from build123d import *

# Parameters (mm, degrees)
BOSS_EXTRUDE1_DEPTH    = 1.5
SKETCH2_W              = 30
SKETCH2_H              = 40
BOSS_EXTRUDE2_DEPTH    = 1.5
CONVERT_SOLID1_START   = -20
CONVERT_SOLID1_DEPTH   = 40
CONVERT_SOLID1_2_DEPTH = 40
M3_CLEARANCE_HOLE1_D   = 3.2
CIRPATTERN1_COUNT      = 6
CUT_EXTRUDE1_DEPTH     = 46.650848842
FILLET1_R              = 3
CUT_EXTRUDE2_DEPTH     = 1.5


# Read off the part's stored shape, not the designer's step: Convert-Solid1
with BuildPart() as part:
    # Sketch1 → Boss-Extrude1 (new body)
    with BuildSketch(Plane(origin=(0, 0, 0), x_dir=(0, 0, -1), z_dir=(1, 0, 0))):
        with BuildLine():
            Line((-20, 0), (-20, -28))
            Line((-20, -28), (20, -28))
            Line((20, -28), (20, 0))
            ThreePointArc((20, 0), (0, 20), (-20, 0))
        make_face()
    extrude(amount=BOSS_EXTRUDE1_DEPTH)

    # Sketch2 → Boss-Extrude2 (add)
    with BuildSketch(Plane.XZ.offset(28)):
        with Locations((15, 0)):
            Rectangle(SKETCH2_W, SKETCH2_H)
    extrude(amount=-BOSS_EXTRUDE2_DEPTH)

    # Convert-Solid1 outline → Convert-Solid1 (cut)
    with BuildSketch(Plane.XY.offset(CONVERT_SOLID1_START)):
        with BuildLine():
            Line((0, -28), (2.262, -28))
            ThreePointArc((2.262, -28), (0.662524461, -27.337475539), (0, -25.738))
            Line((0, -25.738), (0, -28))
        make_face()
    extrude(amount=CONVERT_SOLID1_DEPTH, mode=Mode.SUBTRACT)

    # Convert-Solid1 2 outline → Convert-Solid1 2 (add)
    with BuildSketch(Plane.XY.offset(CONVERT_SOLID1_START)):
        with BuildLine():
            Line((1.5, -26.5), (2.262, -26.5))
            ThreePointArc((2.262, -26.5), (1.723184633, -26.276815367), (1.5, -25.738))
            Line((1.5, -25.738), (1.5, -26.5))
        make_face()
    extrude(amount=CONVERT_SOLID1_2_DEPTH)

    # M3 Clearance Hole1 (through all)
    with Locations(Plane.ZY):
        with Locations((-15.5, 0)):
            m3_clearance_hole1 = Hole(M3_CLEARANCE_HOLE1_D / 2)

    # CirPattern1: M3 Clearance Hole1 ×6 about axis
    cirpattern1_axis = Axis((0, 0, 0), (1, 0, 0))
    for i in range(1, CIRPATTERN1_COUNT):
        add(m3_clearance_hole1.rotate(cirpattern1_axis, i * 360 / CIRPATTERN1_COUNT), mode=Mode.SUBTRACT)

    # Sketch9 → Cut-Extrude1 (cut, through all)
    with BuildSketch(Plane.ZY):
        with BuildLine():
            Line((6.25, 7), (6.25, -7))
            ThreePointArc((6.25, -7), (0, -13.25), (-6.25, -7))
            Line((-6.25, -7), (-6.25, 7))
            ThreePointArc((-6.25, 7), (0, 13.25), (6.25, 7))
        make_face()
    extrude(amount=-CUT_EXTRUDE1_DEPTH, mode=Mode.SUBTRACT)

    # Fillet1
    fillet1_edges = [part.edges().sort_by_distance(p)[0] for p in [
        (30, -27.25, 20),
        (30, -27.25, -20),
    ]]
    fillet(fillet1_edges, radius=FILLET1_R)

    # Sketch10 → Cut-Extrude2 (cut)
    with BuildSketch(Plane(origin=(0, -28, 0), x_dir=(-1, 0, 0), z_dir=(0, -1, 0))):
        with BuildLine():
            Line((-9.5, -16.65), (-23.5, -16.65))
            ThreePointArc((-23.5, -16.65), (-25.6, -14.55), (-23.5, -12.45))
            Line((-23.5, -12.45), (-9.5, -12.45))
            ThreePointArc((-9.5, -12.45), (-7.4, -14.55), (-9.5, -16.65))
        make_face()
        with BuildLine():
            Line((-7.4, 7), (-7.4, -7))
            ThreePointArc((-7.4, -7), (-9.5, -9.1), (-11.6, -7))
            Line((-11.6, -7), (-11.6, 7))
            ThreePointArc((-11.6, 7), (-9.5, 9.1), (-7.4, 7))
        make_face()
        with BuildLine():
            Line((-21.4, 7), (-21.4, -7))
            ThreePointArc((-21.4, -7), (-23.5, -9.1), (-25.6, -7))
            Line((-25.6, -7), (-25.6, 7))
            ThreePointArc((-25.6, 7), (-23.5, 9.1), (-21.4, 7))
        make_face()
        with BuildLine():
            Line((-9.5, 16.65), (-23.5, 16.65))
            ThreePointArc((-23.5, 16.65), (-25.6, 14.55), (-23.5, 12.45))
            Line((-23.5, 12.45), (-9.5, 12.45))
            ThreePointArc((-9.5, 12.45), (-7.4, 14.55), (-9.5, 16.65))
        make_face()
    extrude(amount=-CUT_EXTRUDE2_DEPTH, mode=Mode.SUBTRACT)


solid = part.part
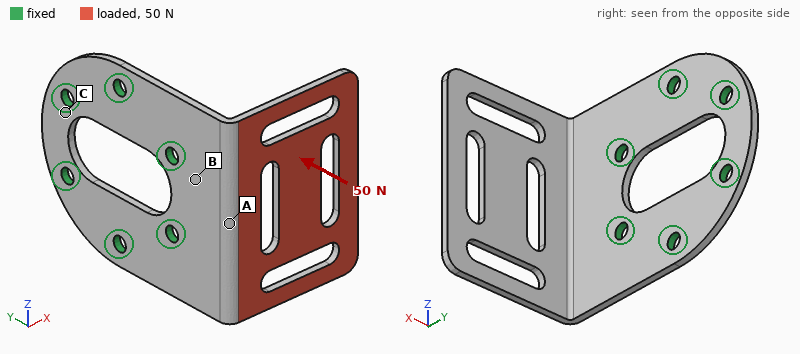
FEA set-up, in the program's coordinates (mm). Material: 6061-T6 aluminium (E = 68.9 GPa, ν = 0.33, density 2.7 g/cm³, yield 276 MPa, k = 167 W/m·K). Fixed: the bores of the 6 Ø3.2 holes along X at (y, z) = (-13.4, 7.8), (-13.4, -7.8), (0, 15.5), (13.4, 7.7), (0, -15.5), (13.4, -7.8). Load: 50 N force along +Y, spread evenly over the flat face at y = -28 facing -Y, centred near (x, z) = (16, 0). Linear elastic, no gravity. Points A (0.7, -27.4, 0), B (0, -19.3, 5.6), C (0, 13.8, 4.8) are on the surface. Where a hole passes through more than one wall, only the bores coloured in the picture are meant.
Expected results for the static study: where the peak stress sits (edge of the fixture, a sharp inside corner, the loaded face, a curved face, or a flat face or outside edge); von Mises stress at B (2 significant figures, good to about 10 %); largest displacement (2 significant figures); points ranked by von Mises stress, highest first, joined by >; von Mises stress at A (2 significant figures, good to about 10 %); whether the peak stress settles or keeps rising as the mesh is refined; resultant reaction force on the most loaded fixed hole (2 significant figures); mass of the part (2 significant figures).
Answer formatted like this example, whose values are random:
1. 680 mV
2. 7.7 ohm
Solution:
1. a sharp inside corner
2. 46 MPa
3. 0.75 mm
4. B > A > C
5. 21 MPa
6. keeps rising
7. 22 N
8. 9.0 g
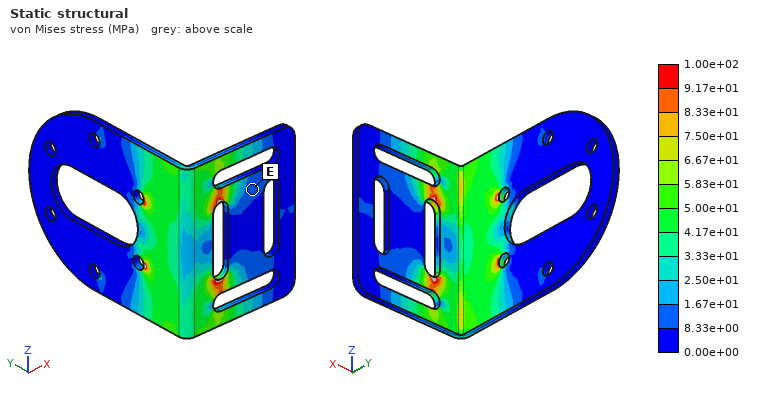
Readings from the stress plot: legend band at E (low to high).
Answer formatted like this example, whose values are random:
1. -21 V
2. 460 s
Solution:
1. 8.33e+00 to 1.67e+01 MPa
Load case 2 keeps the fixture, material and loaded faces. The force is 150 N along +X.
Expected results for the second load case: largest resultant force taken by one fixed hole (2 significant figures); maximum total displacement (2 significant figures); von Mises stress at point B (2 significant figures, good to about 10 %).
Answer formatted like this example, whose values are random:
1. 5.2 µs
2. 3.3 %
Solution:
1. 93 N
2. 0.67 mm
3. 88 MPa
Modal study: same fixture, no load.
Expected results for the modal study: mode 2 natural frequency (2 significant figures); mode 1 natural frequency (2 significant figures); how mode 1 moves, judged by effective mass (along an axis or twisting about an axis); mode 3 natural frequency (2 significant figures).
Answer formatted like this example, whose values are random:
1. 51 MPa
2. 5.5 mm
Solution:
1. 1700 Hz
2. 860 Hz
3. along Y
4. 2600 Hz
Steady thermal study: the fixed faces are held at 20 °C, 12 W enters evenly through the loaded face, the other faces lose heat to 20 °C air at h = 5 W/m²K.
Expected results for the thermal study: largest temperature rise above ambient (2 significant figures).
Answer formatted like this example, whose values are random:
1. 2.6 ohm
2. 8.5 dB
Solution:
1. 57 K
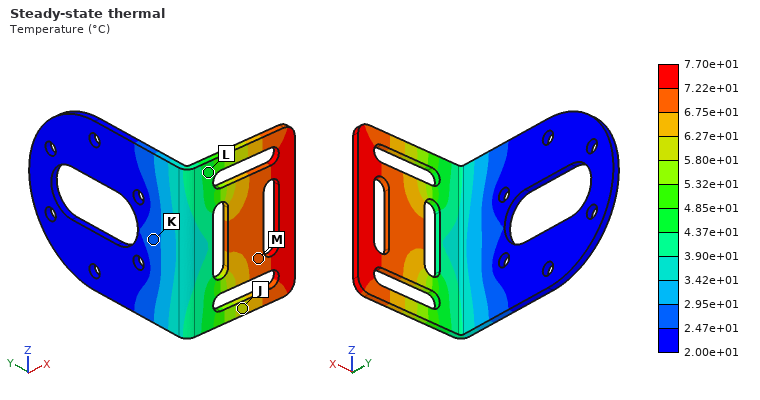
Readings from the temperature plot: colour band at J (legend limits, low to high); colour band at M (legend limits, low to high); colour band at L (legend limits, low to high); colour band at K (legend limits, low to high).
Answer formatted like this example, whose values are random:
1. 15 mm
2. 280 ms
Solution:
1. 5.80e+01 to 6.27e+01 °C
2. 6.75e+01 to 7.22e+01 °C
3. 4.37e+01 to 4.85e+01 °C
4. 2.47e+01 to 2.95e+01 °C
